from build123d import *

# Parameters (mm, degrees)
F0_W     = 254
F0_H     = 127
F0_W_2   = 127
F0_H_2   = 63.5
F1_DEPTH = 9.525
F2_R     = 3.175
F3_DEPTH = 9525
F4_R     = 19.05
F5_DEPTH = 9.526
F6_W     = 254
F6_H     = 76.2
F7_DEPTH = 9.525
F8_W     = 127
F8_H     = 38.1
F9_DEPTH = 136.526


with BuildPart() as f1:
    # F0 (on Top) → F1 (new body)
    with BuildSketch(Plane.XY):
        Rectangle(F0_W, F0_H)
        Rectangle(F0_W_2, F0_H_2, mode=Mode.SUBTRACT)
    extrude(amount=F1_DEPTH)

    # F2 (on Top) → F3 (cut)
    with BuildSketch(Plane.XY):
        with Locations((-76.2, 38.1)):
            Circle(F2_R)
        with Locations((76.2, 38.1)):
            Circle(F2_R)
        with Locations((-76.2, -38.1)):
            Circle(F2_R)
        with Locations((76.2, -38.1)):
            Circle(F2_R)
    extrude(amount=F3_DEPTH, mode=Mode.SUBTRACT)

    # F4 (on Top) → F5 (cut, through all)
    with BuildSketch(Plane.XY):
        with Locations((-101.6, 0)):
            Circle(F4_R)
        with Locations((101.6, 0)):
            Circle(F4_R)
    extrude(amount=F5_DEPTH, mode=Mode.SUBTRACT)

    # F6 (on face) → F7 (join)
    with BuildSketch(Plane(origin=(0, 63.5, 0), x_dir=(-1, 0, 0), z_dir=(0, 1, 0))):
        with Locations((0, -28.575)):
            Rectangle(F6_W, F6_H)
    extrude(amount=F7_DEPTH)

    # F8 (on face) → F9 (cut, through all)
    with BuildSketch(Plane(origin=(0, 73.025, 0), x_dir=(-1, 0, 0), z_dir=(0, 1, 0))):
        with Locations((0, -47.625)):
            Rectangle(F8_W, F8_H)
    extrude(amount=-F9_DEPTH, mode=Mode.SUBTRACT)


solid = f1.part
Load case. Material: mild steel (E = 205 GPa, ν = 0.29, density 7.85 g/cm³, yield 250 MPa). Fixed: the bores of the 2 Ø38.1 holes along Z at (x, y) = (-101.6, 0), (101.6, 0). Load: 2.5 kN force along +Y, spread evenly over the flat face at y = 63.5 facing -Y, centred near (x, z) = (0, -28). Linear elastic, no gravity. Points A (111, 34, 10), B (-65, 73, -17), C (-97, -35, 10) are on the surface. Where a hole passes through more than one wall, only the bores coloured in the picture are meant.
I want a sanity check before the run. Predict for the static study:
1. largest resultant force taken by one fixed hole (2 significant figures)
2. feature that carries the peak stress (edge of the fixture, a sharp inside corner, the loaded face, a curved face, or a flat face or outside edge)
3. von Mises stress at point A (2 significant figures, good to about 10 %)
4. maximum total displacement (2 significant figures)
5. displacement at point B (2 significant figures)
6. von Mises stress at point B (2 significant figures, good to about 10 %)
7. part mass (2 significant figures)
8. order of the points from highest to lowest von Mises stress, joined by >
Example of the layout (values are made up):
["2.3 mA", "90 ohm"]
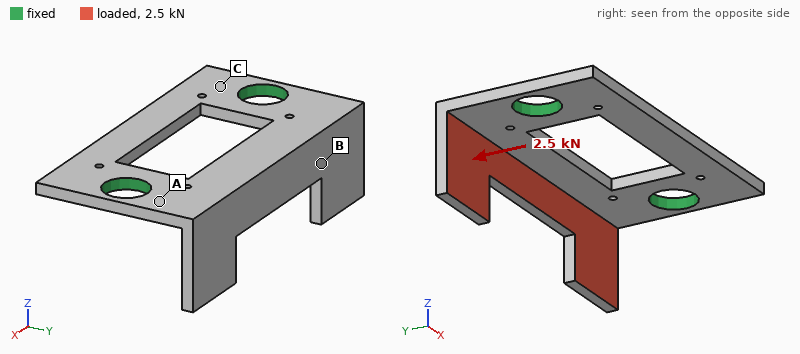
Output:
["1.3 kN", "a curved face", "37 MPa", "0.18 mm", "0.080 mm", "13 MPa", "2.7 kg", "A > B > C"]
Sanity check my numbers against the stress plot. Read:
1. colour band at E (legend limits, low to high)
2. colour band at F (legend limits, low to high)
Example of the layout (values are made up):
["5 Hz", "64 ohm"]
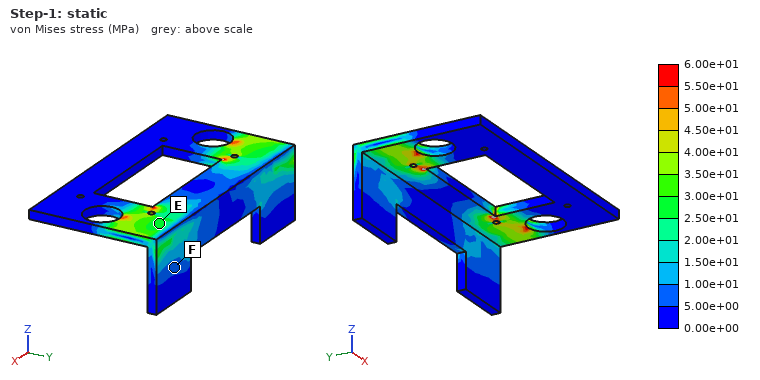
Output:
["2.50e+01 to 3.00e+01 MPa", "5.00e+00 to 1.00e+01 MPa"]
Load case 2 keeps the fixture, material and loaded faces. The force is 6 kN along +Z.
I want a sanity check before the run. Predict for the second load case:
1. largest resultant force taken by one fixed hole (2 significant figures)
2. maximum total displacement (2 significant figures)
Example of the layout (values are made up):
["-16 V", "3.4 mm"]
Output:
["3.0 kN", "0.28 mm"]
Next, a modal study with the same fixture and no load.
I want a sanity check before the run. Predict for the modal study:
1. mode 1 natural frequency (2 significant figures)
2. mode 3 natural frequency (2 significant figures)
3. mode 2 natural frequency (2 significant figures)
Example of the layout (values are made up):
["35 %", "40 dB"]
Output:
["640 Hz", "1300 Hz", "910 Hz"]
